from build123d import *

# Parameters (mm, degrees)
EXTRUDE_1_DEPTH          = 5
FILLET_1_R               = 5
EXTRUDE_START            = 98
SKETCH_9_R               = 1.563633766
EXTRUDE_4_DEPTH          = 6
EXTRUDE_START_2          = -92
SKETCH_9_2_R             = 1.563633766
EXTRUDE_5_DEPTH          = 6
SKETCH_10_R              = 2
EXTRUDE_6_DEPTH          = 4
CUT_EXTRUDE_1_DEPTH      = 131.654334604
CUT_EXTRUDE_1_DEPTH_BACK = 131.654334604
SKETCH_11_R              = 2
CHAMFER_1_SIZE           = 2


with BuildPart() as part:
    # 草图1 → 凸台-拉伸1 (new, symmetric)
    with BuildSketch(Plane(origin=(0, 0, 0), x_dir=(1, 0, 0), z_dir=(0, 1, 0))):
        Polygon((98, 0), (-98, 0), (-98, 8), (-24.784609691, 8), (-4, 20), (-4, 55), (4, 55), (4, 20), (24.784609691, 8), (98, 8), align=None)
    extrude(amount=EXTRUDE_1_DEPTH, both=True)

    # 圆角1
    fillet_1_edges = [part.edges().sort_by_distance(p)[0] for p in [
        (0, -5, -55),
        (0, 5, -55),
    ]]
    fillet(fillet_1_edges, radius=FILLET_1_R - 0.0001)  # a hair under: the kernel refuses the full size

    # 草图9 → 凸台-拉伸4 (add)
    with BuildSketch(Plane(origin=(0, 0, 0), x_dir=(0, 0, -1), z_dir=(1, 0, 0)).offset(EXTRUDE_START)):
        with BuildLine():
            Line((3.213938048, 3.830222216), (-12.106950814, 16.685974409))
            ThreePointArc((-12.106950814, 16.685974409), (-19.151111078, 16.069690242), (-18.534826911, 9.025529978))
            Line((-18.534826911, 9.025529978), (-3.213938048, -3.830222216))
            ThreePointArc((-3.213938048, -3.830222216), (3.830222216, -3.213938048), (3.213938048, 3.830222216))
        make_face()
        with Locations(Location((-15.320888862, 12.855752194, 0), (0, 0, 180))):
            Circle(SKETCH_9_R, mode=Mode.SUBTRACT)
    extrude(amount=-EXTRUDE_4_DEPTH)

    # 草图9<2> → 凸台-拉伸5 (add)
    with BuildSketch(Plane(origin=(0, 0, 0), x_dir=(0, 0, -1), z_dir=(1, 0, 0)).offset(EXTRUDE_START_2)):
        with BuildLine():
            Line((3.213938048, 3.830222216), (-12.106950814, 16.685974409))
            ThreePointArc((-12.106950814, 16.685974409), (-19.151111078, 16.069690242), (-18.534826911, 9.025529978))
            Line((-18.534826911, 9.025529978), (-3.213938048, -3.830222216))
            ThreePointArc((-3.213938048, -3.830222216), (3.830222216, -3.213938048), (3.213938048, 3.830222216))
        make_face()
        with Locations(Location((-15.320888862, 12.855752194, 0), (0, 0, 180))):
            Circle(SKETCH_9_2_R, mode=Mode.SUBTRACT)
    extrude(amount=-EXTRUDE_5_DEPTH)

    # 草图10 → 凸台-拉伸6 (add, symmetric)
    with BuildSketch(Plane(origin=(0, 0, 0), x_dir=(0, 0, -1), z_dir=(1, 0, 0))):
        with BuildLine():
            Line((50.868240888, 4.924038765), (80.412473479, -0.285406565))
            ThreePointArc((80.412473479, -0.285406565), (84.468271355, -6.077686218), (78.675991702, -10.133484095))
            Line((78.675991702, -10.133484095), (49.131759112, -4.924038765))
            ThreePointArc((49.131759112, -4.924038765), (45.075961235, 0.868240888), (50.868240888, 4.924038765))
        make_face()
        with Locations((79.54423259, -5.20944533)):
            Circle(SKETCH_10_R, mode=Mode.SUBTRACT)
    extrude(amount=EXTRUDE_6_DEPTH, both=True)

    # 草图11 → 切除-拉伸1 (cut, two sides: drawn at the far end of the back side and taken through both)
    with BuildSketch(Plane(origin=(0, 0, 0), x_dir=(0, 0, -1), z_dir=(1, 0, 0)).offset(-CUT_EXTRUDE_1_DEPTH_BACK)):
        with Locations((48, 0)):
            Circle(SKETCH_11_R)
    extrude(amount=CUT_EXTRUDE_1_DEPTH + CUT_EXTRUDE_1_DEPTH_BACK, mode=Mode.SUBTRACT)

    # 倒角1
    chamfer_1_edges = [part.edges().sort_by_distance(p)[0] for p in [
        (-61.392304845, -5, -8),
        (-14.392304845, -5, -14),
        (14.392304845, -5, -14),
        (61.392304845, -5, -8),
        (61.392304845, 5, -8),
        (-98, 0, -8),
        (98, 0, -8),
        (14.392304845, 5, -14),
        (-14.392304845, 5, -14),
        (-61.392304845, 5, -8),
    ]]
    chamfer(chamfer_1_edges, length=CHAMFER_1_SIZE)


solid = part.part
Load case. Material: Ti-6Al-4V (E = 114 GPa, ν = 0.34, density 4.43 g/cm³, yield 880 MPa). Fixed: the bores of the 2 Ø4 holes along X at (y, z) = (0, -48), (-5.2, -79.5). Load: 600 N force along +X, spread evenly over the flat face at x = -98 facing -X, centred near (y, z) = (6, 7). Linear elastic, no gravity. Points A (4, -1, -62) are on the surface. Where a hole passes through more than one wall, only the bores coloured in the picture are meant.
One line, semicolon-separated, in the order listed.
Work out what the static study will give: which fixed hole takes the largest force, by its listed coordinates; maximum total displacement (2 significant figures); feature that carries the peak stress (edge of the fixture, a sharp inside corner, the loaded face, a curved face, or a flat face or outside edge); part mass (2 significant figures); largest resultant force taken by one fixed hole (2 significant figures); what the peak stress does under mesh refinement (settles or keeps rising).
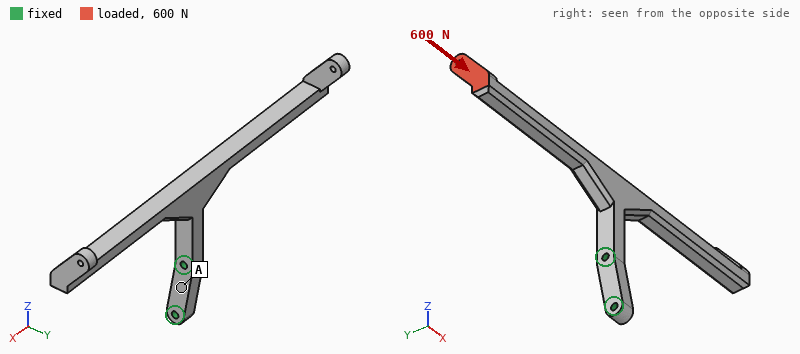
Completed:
(0, -48); 2.3 mm; edge of the fixture; 120 g; 670 N; keeps rising
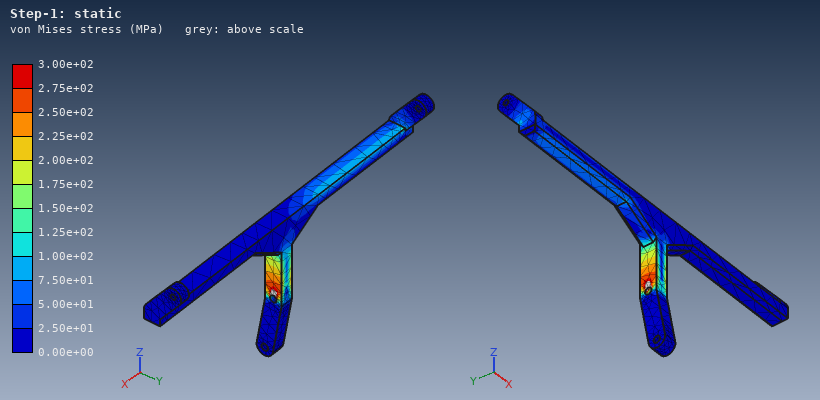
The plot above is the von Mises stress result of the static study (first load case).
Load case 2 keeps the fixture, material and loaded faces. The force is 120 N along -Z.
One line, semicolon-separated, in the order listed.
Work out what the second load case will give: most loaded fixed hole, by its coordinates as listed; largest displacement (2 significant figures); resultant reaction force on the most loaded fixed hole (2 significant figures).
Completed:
(0, -48); 1.4 mm; 120 N
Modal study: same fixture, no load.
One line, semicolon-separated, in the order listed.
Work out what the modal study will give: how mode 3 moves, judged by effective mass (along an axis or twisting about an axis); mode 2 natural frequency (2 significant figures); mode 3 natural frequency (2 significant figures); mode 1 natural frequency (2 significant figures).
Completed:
along Y; 290 Hz; 560 Hz; 290 Hz
